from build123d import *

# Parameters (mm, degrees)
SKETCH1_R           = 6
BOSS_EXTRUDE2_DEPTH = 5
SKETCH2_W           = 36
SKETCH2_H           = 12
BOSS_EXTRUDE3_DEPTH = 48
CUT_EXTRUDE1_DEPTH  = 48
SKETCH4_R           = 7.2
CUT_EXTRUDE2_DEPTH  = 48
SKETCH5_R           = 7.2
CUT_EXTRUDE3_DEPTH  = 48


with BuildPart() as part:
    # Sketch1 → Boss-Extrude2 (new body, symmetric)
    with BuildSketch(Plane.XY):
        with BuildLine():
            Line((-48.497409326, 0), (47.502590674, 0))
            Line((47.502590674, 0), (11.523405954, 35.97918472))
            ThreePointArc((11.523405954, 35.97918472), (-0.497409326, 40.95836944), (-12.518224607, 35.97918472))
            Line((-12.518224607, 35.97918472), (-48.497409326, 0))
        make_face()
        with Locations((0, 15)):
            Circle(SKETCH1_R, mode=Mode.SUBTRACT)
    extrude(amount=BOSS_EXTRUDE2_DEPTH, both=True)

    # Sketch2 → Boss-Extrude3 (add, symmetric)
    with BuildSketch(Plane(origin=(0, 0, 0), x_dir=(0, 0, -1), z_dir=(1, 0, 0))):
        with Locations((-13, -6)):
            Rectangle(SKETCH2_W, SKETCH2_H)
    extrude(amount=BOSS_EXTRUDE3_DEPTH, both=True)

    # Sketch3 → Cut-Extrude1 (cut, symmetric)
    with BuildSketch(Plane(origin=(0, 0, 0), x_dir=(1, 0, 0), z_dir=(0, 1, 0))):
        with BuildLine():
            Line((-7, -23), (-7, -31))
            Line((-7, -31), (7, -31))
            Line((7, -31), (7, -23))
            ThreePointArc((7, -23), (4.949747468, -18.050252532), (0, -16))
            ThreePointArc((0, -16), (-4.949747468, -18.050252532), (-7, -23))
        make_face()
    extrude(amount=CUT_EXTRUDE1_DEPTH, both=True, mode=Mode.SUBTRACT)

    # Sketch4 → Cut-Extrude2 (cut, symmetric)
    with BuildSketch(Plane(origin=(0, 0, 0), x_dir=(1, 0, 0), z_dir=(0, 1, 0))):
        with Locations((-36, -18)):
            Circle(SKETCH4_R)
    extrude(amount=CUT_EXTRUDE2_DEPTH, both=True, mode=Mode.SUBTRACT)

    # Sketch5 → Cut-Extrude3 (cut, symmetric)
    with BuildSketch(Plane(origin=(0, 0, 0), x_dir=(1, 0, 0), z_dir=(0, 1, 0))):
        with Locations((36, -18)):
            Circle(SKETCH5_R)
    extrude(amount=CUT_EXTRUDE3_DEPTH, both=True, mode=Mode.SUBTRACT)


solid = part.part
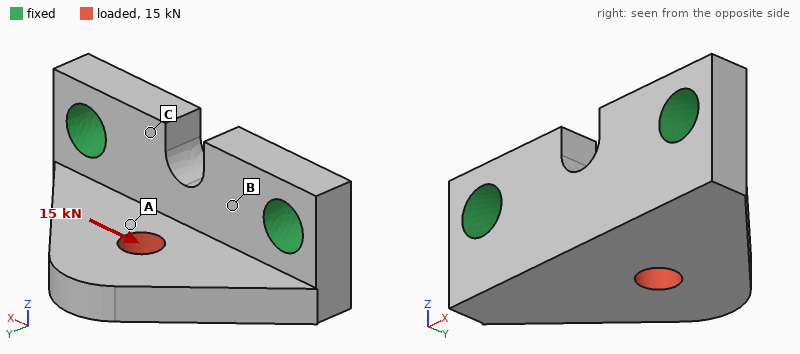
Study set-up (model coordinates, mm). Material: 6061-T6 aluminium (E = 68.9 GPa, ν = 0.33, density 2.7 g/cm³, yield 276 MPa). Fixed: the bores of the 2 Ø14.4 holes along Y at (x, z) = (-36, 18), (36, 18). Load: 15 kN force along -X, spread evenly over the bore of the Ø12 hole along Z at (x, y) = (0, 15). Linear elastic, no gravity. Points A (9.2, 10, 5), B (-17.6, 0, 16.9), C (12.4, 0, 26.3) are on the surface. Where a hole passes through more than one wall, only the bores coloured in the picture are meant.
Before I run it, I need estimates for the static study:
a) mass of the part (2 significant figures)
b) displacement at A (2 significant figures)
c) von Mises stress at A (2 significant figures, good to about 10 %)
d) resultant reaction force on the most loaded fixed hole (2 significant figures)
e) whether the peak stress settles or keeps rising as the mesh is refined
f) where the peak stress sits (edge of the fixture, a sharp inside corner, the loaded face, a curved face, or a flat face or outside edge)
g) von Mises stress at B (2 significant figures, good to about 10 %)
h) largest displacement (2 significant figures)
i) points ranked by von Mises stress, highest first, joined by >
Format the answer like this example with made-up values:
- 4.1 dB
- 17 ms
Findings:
- 150 g
- 28 µm
- 47 MPa
- 9.0 kN
- keeps rising
- edge of the fixture
- 24 MPa
- 47 µm
- A > B > C
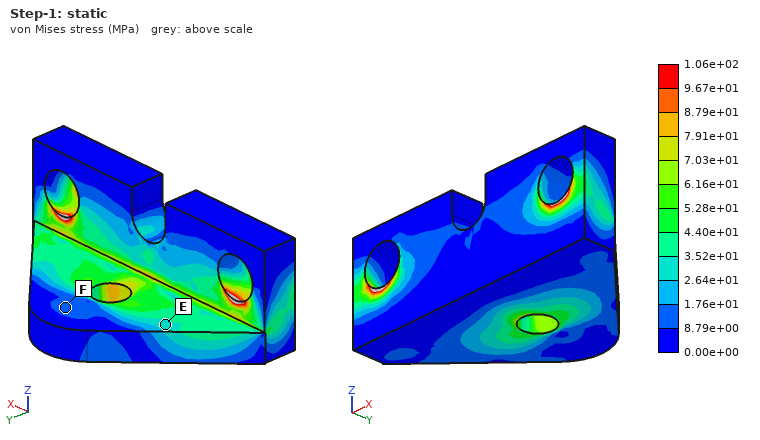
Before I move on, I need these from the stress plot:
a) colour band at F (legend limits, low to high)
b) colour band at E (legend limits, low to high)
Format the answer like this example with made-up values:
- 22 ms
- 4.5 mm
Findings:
- 8.79e+00 to 1.76e+01 MPa
- 2.64e+01 to 3.52e+01 MPa
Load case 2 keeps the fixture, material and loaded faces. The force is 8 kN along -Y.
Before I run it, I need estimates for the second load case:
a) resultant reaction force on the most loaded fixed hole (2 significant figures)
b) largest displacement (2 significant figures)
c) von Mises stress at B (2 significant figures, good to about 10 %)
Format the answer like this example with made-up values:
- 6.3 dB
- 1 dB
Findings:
- 4.1 kN
- 81 µm
- 21 MPa
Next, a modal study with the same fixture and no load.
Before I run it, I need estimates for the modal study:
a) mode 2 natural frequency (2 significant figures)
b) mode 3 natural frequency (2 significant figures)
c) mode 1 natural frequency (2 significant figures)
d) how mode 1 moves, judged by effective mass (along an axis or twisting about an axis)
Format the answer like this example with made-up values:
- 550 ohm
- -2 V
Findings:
- 10 kHz
- 11 kHz
- 4200 Hz
- along Z
